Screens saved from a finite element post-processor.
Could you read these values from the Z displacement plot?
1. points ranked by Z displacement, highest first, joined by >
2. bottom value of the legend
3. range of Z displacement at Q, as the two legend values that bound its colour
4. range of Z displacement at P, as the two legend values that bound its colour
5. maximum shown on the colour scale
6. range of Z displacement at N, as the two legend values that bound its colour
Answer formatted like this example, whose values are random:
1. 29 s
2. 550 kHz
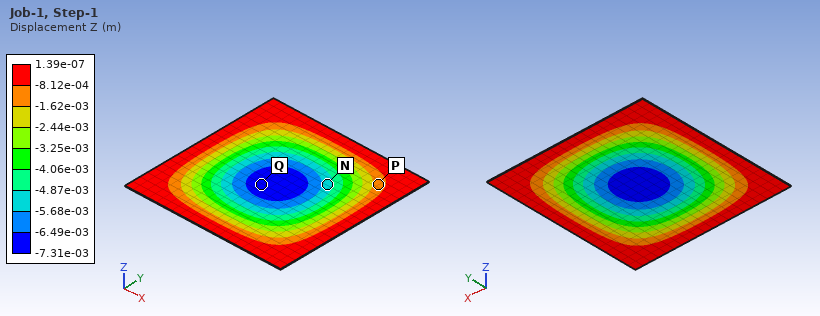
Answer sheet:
1. P > N > Q
2. -7.31e-03 m
3. -7.31e-03 to -6.49e-03 m
4. -1.62e-03 to -8.12e-04 m
5. 1.39e-07 m
6. -5.68e-03 to -4.87e-03 m
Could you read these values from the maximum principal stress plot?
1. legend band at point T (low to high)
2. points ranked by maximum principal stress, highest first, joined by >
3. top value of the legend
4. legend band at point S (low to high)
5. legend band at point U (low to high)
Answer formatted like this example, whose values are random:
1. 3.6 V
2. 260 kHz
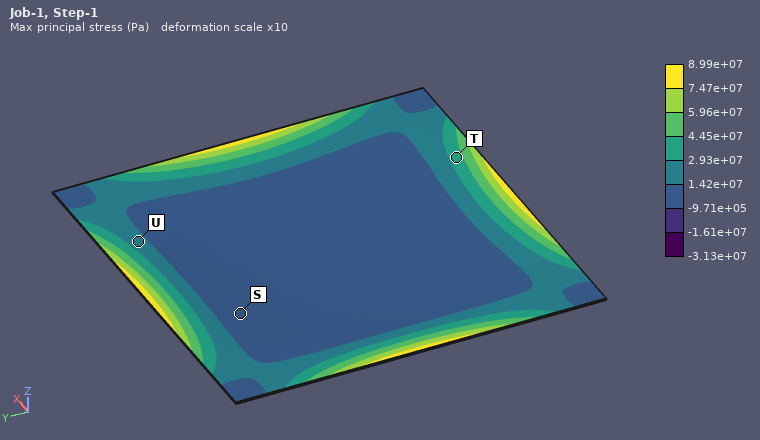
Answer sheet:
1. 2.93e+07 to 4.45e+07 Pa
2. T > U > S
3. 8.99e+07 Pa
4. -9.71e+05 to 1.42e+07 Pa
5. 1.42e+07 to 2.93e+07 Pa
